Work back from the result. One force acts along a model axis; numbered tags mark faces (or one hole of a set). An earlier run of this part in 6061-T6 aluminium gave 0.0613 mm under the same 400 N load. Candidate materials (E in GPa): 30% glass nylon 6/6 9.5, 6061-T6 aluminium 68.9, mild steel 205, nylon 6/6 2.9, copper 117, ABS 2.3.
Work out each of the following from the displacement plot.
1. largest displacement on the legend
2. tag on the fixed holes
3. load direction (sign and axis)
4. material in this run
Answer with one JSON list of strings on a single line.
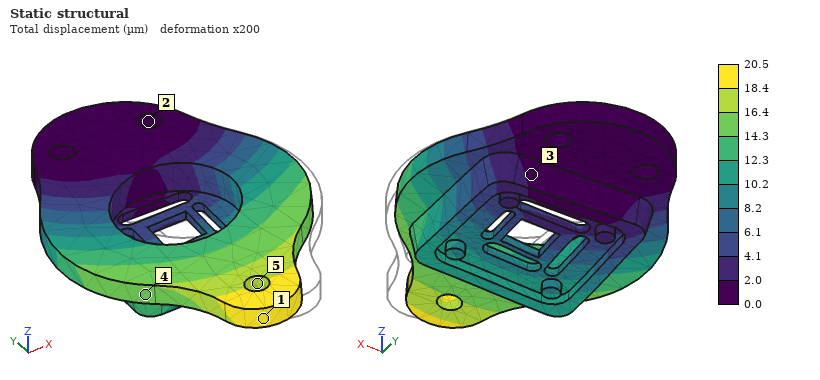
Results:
["20.5 µm", "2", "-X", "mild steel"]
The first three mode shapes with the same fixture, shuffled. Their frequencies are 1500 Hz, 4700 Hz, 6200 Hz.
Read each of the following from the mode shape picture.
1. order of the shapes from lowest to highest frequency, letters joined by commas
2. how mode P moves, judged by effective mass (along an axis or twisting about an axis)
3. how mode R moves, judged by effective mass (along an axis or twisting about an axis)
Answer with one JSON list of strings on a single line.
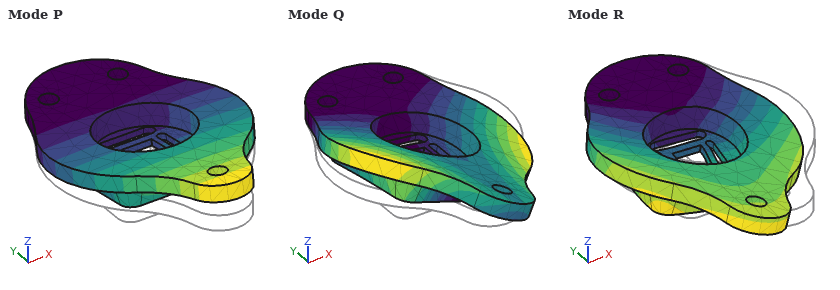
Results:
["P, Q, R", "along Z", "along X"]
